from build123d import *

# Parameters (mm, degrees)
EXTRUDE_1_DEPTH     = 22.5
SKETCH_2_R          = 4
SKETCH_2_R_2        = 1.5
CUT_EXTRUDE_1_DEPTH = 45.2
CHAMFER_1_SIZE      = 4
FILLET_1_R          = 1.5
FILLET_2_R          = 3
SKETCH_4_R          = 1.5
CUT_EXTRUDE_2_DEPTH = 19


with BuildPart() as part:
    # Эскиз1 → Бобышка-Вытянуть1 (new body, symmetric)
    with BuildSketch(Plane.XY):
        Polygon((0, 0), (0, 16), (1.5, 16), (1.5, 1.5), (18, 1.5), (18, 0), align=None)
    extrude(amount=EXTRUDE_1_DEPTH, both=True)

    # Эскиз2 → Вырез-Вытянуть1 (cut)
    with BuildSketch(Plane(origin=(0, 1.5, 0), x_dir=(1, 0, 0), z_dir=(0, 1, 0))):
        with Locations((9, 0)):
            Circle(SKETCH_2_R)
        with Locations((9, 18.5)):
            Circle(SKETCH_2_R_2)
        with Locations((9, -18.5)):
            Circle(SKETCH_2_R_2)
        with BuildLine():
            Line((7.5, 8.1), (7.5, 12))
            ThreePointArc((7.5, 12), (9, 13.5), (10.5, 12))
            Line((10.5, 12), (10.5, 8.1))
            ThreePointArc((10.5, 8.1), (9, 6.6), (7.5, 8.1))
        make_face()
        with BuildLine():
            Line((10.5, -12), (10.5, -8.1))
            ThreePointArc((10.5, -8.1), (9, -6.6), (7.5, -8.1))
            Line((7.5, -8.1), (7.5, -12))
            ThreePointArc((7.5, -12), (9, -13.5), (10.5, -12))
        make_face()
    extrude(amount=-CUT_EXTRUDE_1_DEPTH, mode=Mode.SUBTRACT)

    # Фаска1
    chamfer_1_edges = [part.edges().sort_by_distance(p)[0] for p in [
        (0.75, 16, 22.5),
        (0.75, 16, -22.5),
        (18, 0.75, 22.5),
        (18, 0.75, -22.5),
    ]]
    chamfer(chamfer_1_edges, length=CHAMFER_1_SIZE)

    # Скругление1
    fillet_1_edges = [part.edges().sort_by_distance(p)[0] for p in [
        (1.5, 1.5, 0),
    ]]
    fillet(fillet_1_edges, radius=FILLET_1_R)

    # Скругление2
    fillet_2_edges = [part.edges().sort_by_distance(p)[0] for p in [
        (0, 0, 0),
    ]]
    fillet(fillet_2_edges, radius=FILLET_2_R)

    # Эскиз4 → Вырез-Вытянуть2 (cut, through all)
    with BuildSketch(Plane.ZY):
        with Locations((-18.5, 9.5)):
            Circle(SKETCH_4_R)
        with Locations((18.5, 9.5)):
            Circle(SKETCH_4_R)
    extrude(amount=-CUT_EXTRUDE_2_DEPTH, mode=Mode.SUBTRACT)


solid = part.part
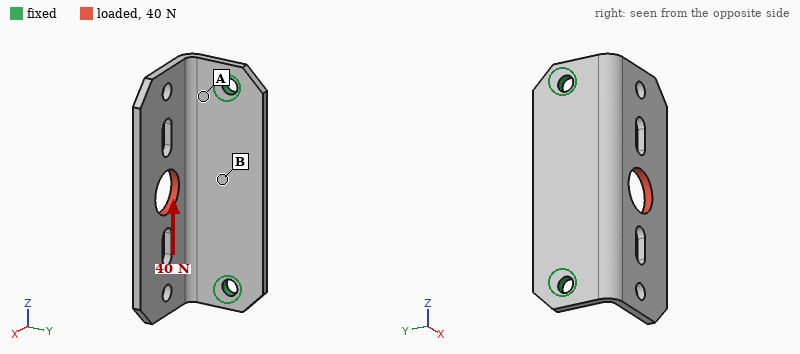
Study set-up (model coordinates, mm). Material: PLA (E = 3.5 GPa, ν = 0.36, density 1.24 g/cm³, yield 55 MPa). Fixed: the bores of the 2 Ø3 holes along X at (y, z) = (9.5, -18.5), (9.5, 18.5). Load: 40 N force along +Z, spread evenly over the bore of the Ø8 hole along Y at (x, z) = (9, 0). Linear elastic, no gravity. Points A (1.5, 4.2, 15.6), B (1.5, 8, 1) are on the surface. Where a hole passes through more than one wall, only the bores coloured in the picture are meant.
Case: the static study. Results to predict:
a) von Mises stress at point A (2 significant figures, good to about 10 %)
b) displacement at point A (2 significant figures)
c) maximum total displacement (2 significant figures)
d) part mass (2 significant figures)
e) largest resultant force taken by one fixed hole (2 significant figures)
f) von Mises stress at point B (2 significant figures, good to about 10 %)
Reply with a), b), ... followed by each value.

a) 5.3 MPa
b) 0.036 mm
c) 0.21 mm
d) 2.4 g
e) 24 N
f) 2.0 MPa
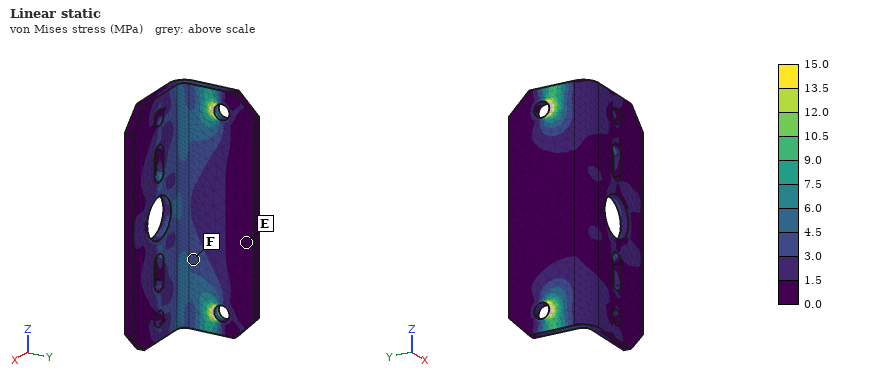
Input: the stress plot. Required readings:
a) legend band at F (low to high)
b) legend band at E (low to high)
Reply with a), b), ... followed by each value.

a) 3.0 to 4.5 MPa
b) 0.0 to 1.5 MPa
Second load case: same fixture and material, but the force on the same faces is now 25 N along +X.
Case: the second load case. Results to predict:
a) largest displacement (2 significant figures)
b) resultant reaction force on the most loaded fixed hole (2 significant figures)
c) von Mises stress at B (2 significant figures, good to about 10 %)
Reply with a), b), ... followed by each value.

a) 0.51 mm
b) 13 N
c) 1.9 MPa
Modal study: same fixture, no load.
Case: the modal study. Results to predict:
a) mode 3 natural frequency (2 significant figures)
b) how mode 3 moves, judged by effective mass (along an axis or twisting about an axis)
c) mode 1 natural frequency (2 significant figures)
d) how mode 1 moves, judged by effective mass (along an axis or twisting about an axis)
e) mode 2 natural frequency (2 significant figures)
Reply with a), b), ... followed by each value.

a) 2100 Hz
b) along X
c) 750 Hz
d) along Y
e) 1300 Hz
